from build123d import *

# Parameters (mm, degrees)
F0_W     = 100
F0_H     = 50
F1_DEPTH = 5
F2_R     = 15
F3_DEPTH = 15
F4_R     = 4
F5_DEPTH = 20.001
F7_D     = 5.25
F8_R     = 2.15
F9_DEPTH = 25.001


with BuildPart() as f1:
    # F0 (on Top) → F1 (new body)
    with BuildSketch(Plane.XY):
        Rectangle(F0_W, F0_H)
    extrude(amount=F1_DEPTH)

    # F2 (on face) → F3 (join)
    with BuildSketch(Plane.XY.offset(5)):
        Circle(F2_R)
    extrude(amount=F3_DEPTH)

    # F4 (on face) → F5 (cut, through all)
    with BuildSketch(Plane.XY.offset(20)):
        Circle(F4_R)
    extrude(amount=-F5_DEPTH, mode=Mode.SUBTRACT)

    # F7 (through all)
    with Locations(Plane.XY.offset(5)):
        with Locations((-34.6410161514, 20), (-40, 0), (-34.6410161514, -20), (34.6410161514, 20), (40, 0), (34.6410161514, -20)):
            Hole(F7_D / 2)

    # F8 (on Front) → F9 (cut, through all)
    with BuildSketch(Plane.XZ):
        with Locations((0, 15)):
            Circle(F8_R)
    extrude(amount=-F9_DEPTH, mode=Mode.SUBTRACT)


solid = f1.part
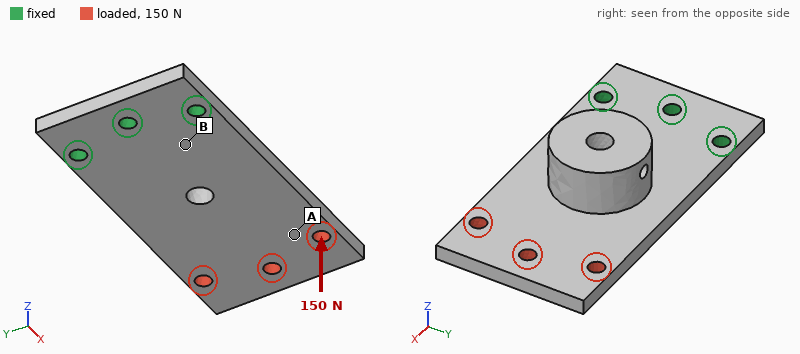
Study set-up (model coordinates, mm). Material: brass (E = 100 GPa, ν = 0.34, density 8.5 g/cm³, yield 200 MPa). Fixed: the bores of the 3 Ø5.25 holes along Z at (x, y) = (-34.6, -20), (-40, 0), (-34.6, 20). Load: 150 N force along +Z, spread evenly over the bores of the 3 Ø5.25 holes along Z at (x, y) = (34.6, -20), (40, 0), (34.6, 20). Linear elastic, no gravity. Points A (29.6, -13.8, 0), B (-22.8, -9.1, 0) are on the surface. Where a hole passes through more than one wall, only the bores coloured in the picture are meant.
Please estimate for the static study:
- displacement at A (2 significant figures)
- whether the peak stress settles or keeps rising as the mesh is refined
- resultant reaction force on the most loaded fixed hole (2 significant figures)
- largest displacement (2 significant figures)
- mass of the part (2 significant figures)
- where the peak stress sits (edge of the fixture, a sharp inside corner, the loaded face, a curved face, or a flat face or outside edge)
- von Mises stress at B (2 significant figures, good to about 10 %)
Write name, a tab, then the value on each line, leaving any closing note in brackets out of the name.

displacement at A	0.23 mm
whether the peak stress settles or keeps rising as the mesh is refined	keeps rising
resultant reaction force on the most loaded fixed hole	140 N
largest displacement	0.33 mm
mass of the part	290 g
where the peak stress sits	edge of the fixture
von Mises stress at B	37 MPa
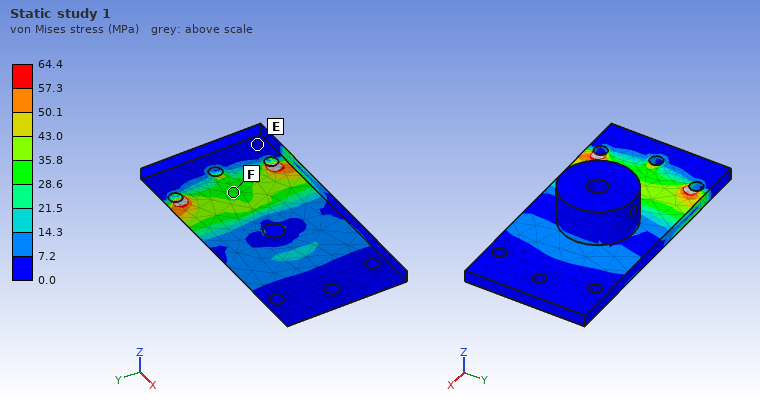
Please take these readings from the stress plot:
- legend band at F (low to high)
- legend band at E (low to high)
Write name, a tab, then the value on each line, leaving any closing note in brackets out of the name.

legend band at F	28.6 to 35.8 MPa
legend band at E	0.0 to 7.2 MPa
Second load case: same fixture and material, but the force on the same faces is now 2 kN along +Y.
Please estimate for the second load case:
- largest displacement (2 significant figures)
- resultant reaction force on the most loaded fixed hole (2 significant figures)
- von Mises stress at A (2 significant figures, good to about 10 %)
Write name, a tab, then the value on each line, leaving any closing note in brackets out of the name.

largest displacement	80 µm
resultant reaction force on the most loaded fixed hole	3.5 kN
von Mises stress at A	17 MPa
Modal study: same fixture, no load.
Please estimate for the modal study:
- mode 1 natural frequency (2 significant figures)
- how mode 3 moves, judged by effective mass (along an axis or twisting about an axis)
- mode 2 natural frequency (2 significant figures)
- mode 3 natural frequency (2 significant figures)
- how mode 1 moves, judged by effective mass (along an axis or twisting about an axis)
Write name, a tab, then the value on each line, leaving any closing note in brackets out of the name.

mode 1 natural frequency	410 Hz
how mode 3 moves, judged by effective mass	along Z
mode 2 natural frequency	1800 Hz
mode 3 natural frequency	2400 Hz
how mode 1 moves, judged by effective mass	along Z
